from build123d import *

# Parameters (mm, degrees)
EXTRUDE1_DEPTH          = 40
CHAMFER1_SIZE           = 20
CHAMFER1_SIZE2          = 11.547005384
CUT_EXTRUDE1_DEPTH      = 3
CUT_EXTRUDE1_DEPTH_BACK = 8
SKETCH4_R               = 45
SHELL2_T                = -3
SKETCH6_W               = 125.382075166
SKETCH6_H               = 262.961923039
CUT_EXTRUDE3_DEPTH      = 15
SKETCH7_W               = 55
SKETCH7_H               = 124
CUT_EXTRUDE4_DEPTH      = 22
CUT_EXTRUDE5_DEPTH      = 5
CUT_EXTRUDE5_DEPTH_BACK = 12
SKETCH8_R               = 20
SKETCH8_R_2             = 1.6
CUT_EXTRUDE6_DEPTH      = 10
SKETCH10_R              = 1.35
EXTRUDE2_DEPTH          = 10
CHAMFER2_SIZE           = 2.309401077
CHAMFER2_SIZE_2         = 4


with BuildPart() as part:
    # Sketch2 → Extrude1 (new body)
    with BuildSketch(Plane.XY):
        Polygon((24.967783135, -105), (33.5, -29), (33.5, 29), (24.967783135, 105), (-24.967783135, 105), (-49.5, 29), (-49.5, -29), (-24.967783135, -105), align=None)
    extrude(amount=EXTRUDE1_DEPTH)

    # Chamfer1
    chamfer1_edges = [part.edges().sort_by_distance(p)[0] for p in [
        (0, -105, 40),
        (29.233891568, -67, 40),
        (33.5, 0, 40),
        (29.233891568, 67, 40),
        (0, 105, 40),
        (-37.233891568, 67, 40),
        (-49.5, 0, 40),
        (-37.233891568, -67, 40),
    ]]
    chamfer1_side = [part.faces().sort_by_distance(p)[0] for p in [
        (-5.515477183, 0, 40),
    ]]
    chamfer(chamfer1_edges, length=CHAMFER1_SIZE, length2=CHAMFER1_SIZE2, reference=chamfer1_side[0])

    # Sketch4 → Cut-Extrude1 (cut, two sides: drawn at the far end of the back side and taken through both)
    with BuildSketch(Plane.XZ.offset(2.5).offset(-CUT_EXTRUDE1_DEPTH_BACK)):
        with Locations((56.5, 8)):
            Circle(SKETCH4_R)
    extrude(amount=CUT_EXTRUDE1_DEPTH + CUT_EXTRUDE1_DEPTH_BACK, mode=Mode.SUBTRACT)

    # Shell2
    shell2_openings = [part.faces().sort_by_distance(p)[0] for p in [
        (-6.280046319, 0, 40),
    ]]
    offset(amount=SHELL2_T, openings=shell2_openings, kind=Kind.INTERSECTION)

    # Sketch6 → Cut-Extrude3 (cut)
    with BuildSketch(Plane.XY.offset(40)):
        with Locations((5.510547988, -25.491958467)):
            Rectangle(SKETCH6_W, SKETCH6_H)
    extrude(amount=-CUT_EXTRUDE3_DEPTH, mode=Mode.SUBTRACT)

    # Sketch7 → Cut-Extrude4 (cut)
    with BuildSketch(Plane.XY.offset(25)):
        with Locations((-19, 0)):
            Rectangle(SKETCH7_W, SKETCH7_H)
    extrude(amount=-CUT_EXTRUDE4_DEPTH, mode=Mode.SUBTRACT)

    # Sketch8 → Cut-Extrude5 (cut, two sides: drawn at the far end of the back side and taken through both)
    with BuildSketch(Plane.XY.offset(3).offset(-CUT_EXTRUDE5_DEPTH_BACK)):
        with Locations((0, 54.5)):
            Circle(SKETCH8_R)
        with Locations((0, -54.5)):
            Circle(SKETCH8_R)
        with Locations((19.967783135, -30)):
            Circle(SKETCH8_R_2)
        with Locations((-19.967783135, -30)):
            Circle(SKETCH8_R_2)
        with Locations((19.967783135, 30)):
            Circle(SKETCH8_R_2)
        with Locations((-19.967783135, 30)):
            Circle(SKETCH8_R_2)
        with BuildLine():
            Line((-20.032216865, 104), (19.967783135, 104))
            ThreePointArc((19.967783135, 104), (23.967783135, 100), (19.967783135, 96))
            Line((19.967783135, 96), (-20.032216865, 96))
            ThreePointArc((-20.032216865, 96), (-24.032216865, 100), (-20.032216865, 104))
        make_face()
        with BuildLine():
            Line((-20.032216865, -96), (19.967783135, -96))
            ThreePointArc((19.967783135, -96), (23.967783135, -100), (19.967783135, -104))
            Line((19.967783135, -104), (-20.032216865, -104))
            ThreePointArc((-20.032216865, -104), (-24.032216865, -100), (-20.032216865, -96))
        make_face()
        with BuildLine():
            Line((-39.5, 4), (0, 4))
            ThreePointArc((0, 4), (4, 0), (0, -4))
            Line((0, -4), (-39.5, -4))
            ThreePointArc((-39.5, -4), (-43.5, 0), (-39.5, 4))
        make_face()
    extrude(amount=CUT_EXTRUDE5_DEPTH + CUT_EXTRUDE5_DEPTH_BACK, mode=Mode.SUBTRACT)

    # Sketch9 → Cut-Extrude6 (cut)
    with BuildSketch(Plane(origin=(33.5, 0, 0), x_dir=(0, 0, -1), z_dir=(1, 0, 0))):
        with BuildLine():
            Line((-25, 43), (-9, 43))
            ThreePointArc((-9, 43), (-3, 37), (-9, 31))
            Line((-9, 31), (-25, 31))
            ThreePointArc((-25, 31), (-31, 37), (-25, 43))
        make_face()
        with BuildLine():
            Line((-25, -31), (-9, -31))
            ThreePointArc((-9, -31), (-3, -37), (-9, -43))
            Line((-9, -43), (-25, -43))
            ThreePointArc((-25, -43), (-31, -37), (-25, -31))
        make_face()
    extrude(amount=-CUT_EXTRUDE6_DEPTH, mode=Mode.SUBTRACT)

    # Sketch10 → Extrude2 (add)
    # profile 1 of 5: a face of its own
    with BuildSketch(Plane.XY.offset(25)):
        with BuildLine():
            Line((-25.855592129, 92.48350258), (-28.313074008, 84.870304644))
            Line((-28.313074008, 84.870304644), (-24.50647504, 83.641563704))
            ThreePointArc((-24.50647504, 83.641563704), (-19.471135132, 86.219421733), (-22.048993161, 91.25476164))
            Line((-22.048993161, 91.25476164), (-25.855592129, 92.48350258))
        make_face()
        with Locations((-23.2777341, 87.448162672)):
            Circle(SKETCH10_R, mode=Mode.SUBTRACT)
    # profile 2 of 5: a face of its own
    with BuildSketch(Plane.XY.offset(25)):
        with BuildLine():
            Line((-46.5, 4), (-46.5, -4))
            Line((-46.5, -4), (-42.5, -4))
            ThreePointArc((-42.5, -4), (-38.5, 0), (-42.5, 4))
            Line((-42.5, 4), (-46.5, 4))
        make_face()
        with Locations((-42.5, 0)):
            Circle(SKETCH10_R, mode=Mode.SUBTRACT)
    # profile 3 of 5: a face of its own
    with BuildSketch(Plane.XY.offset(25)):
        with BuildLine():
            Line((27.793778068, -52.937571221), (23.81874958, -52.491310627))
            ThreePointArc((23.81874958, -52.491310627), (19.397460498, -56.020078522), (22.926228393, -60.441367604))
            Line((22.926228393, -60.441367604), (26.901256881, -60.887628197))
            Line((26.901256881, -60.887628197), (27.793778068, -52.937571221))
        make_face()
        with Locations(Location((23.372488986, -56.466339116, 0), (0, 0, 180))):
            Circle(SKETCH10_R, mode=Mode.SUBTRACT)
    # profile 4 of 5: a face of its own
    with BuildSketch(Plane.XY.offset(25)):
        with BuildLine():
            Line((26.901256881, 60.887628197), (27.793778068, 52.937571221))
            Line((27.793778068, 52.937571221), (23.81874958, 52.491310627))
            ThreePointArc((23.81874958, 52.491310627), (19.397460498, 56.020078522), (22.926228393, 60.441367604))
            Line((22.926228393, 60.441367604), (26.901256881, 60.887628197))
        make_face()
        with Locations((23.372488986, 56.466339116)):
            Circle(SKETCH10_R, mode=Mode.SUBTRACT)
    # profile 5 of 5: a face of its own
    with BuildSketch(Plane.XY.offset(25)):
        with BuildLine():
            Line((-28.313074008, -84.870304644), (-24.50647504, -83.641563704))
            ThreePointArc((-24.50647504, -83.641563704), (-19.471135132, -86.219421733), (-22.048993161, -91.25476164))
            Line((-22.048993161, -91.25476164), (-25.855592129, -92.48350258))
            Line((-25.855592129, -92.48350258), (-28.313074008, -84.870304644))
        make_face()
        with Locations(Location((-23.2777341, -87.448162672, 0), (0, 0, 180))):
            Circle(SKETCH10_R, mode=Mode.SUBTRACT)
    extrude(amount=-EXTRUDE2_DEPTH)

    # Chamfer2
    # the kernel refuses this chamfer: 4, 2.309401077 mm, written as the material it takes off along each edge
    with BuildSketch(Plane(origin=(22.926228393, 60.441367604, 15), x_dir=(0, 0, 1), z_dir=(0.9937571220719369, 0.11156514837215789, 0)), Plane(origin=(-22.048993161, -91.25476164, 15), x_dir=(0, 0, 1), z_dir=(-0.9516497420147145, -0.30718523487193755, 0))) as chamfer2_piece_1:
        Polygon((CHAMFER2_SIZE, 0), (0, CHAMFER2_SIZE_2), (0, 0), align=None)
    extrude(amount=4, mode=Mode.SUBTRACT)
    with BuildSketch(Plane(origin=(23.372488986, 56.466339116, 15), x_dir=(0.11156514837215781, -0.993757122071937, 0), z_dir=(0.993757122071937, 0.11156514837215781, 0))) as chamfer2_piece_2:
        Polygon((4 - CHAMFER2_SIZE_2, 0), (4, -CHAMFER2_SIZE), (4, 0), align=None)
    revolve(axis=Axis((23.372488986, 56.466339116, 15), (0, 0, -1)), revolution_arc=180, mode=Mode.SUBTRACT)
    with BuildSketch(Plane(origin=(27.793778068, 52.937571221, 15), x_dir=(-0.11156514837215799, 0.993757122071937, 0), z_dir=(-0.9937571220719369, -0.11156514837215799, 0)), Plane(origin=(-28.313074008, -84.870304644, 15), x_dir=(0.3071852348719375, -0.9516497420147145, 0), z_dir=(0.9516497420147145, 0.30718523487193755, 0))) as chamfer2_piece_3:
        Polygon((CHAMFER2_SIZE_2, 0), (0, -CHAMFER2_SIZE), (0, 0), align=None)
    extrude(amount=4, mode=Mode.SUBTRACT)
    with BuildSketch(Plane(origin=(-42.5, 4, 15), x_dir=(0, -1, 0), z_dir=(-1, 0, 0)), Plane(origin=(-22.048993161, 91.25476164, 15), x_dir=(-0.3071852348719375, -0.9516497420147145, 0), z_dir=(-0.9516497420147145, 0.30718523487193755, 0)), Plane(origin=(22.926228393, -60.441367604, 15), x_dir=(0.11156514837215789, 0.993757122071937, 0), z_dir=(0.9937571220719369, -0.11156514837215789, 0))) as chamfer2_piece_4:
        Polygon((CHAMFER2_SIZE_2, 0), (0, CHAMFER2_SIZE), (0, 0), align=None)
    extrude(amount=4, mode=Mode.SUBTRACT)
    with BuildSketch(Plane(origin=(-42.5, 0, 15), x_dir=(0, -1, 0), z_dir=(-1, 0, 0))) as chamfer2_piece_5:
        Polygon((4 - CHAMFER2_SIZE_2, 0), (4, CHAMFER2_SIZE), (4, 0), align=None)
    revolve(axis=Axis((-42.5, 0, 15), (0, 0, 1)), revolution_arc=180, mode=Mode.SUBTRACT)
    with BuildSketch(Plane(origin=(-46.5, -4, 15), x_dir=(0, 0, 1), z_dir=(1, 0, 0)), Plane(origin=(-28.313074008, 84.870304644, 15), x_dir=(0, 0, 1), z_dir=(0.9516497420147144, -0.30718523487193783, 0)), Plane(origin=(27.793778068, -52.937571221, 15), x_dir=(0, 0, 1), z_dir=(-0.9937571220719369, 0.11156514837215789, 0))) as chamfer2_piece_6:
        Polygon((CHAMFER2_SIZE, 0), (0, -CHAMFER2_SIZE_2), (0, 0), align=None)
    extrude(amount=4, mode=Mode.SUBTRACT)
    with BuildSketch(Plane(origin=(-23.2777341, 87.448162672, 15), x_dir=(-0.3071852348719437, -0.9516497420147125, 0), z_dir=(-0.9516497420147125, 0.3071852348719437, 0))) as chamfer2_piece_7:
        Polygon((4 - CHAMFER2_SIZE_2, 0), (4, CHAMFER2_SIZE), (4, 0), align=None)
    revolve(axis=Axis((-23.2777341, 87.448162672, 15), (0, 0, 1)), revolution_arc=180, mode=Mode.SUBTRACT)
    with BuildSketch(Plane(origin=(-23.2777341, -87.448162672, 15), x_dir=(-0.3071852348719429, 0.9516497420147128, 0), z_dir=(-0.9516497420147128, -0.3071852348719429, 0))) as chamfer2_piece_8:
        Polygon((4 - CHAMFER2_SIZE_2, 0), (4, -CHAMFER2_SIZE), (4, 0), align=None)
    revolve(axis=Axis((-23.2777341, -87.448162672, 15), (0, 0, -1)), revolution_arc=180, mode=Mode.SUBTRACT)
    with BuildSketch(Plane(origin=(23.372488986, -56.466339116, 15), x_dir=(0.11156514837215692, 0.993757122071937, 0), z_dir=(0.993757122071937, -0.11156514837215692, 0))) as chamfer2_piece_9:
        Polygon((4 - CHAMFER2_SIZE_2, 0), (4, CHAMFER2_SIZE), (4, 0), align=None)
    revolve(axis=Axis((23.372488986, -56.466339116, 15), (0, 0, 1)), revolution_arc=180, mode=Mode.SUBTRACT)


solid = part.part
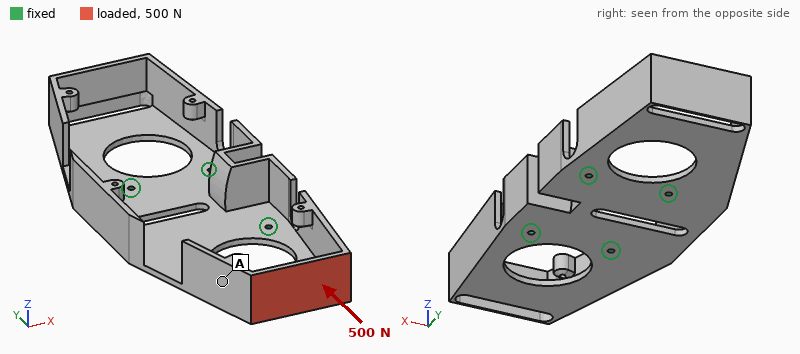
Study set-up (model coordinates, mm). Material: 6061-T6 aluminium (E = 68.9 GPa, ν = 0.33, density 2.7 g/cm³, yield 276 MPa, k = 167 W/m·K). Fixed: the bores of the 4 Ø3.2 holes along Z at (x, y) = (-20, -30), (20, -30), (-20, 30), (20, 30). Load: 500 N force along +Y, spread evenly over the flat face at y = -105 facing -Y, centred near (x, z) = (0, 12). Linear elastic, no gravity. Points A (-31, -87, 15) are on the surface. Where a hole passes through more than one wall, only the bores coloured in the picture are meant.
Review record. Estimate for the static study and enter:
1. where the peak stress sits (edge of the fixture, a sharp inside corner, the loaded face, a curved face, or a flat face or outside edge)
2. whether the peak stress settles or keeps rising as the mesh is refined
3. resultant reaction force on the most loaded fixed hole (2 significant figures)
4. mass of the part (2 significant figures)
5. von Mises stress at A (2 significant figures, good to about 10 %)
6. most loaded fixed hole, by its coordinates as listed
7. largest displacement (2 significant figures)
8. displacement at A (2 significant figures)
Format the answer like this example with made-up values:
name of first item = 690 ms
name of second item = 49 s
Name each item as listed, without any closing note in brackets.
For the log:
where the peak stress sits = a sharp inside corner
whether the peak stress settles or keeps rising as the mesh is refined = keeps rising
resultant reaction force on the most loaded fixed hole = 280 N
mass of the part = 180 g
von Mises stress at A = 12 MPa
most loaded fixed hole, by its coordinates as listed = (20, -30)
largest displacement = 1.2 mm
displacement at A = 0.73 mm
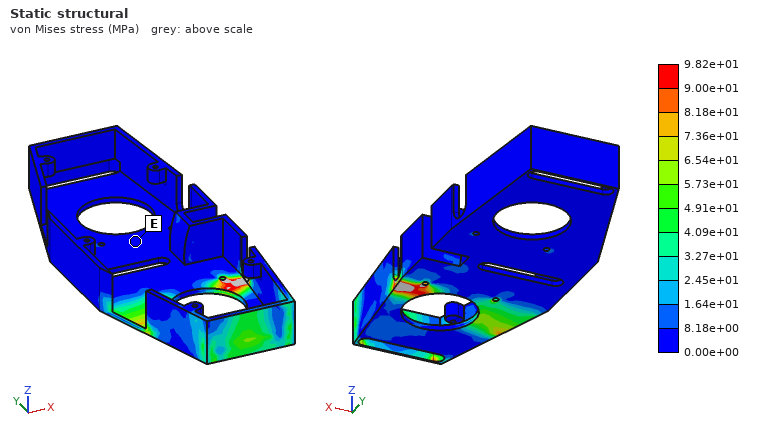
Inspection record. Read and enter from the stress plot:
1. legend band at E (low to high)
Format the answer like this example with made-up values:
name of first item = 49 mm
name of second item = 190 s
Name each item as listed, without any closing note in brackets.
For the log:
legend band at E = 0.00e+00 to 8.18e+00 MPa
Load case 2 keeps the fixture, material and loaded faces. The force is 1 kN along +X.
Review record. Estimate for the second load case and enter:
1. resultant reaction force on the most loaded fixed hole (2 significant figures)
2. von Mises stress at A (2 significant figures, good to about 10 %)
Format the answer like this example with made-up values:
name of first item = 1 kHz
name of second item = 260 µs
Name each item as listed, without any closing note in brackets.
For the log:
resultant reaction force on the most loaded fixed hole = 1.3 kN
von Mises stress at A = 29 MPa
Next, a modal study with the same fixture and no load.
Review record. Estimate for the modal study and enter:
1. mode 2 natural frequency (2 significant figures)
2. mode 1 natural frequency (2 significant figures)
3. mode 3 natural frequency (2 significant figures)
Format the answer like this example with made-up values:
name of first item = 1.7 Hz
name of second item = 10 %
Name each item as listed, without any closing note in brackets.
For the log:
mode 2 natural frequency = 300 Hz
mode 1 natural frequency = 300 Hz
mode 3 natural frequency = 830 Hz
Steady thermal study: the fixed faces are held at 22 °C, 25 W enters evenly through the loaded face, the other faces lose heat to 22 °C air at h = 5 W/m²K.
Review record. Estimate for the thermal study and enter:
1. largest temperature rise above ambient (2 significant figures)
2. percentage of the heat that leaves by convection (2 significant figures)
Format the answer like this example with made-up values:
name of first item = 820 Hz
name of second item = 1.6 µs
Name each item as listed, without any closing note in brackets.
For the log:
largest temperature rise above ambient = 84 K
percentage of the heat that leaves by convection = 13 %
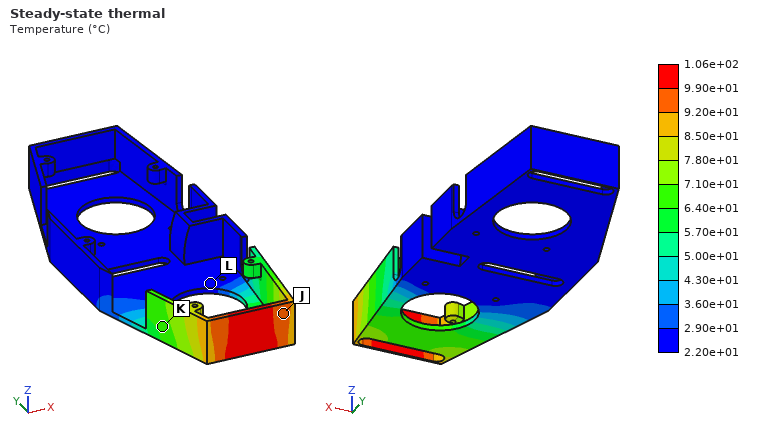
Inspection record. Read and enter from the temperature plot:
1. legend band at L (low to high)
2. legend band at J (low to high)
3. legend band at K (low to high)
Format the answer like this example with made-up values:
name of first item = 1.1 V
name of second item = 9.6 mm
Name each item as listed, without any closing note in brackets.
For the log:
legend band at L = 2.20e+01 to 2.90e+01 °C
legend band at J = 9.20e+01 to 9.90e+01 °C
legend band at K = 6.40e+01 to 7.10e+01 °C
